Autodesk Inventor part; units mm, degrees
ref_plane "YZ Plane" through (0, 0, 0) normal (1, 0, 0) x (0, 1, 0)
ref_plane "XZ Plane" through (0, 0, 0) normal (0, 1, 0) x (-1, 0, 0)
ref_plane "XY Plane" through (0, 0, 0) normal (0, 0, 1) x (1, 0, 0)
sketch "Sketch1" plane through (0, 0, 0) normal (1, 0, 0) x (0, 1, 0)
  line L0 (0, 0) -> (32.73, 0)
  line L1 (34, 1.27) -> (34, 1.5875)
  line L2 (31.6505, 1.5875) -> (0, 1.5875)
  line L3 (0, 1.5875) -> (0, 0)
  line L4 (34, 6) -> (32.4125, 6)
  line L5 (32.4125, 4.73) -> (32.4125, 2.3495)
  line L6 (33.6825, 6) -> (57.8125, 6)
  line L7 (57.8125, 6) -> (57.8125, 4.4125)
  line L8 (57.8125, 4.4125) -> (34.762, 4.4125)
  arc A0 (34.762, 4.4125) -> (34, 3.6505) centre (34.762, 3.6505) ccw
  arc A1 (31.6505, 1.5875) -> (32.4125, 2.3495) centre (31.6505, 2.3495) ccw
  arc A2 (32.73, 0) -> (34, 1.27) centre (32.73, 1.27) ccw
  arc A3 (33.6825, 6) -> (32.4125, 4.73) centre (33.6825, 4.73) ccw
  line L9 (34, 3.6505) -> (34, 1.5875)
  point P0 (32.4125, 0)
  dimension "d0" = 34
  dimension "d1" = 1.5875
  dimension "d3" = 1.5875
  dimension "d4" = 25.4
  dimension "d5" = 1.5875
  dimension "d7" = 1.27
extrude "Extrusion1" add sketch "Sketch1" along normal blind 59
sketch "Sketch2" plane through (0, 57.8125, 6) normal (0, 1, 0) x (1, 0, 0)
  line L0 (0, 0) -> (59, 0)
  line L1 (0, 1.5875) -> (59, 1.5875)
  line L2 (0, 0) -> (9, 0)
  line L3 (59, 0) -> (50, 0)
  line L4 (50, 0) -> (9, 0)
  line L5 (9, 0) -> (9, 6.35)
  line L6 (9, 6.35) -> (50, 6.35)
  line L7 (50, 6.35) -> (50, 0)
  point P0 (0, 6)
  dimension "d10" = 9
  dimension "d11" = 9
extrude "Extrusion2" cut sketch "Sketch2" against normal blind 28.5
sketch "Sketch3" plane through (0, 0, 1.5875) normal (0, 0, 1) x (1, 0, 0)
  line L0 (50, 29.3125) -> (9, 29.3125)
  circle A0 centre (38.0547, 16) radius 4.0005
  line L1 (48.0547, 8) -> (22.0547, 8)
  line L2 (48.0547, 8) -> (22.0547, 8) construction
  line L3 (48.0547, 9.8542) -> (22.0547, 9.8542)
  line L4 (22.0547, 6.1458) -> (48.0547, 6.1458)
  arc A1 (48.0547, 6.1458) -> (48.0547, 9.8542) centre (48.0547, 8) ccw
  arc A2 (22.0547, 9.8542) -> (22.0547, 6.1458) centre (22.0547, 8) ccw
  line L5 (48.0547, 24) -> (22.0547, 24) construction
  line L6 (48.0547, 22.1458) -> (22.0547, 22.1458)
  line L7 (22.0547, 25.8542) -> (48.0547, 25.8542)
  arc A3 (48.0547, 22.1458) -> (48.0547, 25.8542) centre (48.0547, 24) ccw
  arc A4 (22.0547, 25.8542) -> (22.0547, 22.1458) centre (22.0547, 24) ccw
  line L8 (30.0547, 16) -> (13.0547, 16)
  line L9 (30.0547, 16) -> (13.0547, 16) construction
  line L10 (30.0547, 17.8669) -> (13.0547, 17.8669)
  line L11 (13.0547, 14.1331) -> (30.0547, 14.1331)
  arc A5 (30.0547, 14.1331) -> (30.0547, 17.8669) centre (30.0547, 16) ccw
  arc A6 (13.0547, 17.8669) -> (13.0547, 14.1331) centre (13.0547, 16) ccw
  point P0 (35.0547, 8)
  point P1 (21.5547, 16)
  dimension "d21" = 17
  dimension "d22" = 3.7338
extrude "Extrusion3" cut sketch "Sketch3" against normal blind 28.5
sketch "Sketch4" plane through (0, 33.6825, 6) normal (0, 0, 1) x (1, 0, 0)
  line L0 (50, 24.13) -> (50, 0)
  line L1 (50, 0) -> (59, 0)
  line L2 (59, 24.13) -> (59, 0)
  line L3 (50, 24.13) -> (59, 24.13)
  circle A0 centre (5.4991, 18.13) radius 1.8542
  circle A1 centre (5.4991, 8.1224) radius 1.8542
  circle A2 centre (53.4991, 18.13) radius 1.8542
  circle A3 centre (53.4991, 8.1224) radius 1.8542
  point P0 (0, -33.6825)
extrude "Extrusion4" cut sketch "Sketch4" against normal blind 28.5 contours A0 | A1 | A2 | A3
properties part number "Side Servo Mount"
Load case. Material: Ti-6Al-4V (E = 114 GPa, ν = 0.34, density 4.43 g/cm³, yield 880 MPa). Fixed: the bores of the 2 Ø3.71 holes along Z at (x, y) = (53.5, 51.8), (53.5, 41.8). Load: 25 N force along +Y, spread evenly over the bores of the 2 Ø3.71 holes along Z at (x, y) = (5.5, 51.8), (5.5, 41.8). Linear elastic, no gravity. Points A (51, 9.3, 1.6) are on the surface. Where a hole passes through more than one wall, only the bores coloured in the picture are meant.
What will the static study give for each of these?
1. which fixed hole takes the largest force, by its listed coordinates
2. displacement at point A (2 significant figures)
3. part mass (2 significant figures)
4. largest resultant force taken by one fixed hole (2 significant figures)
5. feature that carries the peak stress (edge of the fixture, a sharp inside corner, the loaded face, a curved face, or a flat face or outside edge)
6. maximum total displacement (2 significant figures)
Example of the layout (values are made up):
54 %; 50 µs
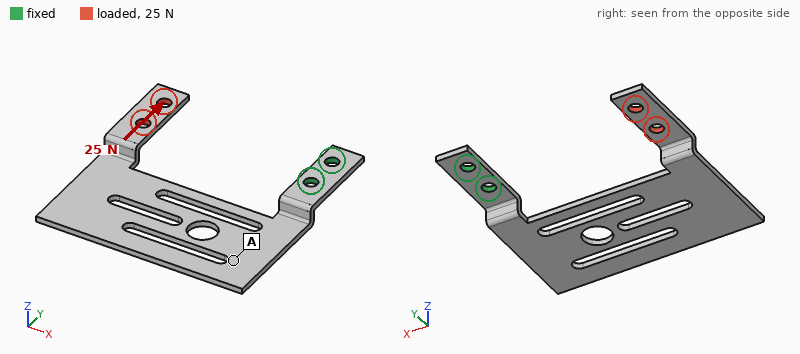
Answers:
(53.5, 41.8); 0.18 mm; 14 g; 76 N; a curved face; 0.84 mm
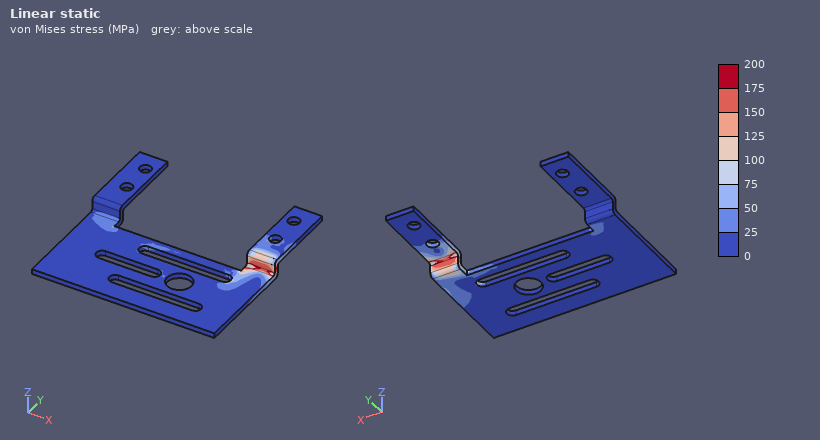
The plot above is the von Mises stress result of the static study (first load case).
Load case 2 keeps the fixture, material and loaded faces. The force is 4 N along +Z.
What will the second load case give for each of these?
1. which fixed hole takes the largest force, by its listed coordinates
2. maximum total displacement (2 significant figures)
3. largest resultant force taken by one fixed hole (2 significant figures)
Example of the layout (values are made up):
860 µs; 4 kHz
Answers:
(53.5, 41.8); 0.94 mm; 2.3 N
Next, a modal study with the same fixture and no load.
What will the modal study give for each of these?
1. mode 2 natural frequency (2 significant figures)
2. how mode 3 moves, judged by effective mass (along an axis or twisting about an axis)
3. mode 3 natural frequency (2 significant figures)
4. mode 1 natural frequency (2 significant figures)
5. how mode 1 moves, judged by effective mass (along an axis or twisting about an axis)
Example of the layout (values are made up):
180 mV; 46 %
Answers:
320 Hz; along Y; 480 Hz; 180 Hz; along Z
